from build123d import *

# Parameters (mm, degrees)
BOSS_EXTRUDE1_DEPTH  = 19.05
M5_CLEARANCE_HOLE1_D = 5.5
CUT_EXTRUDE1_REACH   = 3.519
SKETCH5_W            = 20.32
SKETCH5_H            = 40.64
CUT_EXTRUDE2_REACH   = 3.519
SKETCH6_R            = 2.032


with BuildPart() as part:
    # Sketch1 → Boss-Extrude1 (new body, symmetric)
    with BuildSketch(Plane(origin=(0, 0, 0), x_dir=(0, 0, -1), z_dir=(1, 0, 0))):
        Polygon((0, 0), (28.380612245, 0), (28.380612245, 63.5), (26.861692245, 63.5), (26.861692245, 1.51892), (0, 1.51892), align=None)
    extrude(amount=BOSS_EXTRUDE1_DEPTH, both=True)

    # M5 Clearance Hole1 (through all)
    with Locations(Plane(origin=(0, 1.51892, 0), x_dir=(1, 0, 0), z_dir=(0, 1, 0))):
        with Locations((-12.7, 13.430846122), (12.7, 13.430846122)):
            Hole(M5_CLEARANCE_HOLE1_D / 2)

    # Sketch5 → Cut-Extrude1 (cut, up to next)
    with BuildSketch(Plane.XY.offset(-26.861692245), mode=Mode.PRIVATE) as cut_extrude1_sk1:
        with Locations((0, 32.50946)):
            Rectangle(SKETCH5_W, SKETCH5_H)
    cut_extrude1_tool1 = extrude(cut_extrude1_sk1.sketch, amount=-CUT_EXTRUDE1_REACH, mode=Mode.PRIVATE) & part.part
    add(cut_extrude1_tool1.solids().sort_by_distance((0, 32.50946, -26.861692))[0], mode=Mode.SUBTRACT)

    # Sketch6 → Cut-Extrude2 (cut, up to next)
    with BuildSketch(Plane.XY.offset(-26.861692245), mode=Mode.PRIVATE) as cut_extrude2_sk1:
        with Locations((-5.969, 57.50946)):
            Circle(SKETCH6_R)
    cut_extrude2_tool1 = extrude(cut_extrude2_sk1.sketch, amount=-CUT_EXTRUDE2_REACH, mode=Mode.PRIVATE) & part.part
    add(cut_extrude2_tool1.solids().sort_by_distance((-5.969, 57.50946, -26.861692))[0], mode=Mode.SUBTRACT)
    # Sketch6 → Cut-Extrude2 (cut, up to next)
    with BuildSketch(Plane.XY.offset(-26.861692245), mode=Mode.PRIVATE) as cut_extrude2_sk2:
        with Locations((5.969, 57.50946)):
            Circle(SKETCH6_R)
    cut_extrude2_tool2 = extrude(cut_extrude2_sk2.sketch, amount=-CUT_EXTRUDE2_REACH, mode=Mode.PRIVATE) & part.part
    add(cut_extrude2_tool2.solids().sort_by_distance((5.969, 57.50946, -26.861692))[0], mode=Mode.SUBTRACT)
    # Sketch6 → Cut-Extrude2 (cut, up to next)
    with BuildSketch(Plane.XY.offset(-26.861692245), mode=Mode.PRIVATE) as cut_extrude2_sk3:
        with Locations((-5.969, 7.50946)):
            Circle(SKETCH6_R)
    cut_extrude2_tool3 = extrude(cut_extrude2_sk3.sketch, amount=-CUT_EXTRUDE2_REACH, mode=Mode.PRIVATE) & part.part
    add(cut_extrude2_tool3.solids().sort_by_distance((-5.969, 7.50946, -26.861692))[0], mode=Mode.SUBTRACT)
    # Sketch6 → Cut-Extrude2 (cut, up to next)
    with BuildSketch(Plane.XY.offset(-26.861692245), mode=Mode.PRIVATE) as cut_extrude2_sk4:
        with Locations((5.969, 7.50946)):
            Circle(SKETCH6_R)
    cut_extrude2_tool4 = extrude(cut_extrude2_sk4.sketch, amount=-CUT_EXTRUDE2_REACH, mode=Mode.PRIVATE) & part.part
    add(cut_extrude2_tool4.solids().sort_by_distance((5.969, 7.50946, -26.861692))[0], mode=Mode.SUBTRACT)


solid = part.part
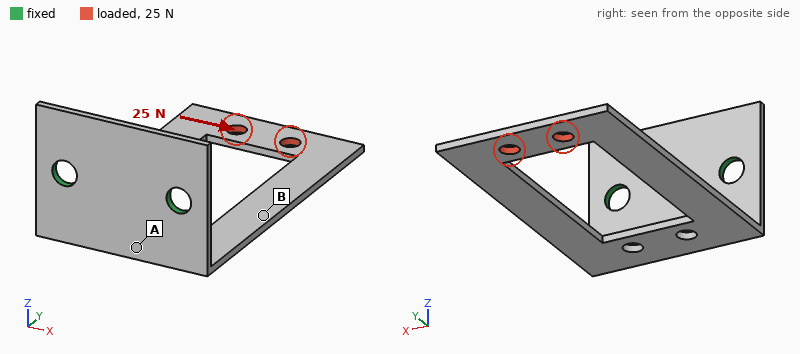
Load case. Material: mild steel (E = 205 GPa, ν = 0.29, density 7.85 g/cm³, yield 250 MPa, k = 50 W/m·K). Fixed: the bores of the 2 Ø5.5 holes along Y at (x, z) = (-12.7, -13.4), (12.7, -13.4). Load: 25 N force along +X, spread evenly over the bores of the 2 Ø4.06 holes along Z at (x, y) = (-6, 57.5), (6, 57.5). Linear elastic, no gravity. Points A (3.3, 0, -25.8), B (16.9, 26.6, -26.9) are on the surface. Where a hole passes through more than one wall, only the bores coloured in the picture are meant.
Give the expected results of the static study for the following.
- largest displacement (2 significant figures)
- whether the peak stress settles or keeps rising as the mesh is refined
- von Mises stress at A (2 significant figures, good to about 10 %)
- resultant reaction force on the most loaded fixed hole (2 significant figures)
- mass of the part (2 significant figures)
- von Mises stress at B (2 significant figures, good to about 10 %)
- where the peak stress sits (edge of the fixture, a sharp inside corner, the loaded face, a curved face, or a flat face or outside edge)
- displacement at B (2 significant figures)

0.10 mm
keeps rising
27 MPa
54 N
30 g
9.1 MPa
edge of the fixture
0.049 mm
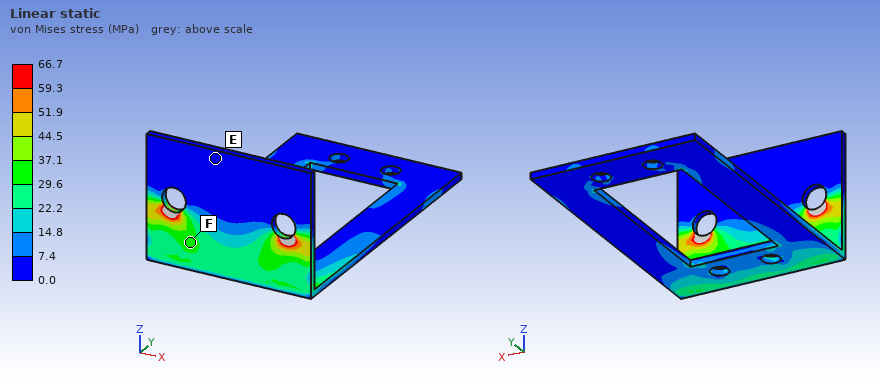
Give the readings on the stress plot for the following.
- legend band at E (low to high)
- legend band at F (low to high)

0.0 to 7.4 MPa
29.6 to 37.1 MPa
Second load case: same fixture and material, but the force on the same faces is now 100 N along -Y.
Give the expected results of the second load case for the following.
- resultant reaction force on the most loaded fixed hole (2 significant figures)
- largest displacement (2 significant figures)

50 N
0.22 mm
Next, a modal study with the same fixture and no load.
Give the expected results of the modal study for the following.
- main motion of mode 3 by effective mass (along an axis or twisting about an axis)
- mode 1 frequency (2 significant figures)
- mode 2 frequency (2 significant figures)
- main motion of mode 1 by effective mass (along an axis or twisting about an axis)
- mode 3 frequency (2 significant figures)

along X
240 Hz
780 Hz
along Z
1000 Hz
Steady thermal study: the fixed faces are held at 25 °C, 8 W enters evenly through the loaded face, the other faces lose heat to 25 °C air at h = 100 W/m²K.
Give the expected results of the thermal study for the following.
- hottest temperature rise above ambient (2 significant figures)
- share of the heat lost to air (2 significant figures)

76 K
98 %
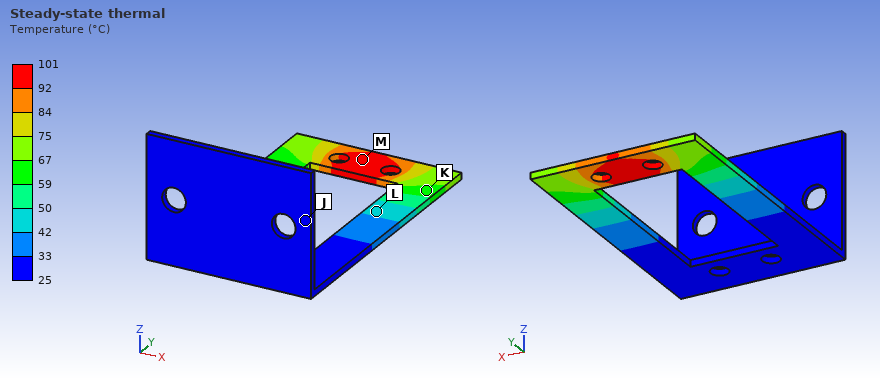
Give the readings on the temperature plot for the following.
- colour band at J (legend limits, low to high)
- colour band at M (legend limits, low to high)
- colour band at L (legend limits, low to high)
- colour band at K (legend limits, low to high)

25 to 33 °C
92 to 101 °C
42 to 50 °C
59 to 67 °C
